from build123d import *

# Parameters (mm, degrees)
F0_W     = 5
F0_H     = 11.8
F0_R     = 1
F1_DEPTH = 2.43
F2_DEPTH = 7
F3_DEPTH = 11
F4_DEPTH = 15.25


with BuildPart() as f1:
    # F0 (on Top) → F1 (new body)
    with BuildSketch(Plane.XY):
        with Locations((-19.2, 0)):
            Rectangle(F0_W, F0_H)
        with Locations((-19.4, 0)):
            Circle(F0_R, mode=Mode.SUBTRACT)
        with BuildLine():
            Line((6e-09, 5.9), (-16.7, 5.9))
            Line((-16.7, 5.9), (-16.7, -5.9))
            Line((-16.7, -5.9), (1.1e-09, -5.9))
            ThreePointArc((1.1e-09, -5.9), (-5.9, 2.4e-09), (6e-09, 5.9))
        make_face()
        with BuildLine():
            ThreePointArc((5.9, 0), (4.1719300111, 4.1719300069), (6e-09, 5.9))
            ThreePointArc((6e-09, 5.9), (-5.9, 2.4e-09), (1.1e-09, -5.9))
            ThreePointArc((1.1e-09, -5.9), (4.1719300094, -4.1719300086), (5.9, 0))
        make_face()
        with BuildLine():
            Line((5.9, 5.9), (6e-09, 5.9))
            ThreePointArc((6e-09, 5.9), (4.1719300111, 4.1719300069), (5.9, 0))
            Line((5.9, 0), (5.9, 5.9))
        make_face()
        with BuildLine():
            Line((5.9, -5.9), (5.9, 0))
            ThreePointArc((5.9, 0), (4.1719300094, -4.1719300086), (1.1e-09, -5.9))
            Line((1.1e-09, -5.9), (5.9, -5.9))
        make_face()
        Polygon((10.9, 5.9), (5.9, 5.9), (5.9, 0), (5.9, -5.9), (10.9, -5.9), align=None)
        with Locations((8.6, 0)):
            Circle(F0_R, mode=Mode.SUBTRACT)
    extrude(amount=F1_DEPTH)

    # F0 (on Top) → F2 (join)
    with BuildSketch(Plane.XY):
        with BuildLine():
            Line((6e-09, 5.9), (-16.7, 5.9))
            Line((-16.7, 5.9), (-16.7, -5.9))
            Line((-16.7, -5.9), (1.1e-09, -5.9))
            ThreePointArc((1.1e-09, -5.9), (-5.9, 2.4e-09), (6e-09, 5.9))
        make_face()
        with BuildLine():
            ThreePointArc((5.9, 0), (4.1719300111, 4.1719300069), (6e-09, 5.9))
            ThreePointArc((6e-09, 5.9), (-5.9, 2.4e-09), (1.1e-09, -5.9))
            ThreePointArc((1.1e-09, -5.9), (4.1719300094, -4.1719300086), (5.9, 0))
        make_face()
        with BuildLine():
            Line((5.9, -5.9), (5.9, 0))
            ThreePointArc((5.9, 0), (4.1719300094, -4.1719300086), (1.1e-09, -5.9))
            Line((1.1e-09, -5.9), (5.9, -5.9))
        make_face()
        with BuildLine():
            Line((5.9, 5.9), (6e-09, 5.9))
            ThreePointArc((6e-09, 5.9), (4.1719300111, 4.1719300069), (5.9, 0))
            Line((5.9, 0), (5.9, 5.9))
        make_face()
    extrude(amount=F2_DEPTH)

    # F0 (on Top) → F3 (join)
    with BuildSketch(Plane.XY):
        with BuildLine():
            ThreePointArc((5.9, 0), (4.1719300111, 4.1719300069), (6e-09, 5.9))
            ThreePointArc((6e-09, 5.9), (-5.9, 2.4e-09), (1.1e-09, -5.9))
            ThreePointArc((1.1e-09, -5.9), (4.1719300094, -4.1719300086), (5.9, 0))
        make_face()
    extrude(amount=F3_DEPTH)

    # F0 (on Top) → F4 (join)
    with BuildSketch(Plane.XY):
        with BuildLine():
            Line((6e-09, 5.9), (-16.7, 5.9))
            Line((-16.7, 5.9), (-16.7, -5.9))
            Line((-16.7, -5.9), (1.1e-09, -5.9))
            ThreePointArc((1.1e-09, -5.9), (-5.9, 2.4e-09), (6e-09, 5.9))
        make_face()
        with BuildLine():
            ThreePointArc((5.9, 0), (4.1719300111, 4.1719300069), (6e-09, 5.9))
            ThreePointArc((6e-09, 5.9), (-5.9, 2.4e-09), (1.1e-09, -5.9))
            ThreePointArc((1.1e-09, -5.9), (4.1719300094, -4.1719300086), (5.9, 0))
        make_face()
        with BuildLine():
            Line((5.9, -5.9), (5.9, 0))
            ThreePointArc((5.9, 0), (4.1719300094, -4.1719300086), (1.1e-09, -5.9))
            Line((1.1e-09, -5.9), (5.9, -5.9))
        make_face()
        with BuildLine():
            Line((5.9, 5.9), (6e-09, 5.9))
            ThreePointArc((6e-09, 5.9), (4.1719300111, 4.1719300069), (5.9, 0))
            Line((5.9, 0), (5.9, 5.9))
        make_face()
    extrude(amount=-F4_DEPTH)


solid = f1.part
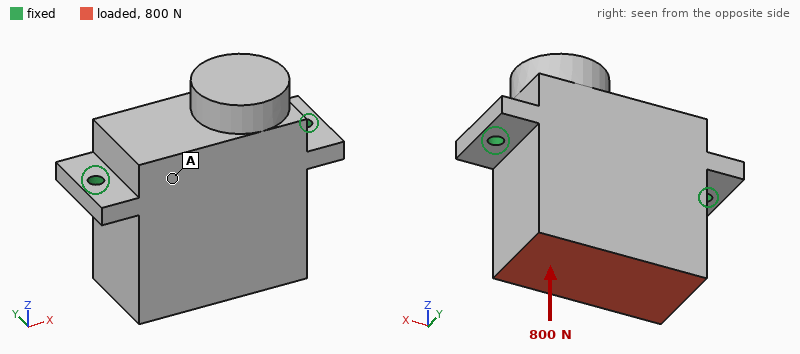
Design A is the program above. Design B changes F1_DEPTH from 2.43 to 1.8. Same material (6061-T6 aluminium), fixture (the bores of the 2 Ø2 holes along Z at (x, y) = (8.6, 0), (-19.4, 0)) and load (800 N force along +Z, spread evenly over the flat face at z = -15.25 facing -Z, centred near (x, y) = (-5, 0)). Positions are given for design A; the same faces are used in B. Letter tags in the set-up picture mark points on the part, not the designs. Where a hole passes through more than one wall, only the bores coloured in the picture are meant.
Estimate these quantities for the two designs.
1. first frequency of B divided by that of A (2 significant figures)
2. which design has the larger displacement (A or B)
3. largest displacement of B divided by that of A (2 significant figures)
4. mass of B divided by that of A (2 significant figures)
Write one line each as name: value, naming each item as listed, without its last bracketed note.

first frequency of B divided by that of A: 0.74
which design has the larger displacement: B
largest displacement of B divided by that of A: 1.4
mass of B divided by that of A: 0.99
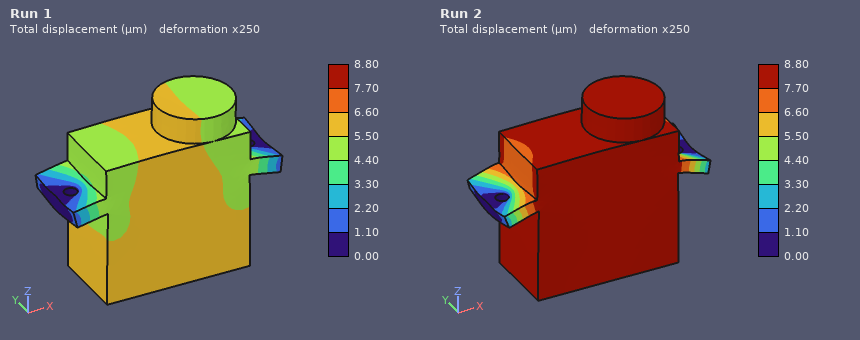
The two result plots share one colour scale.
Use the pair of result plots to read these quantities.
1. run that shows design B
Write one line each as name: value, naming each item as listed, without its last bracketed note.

run that shows design B: Run 2
